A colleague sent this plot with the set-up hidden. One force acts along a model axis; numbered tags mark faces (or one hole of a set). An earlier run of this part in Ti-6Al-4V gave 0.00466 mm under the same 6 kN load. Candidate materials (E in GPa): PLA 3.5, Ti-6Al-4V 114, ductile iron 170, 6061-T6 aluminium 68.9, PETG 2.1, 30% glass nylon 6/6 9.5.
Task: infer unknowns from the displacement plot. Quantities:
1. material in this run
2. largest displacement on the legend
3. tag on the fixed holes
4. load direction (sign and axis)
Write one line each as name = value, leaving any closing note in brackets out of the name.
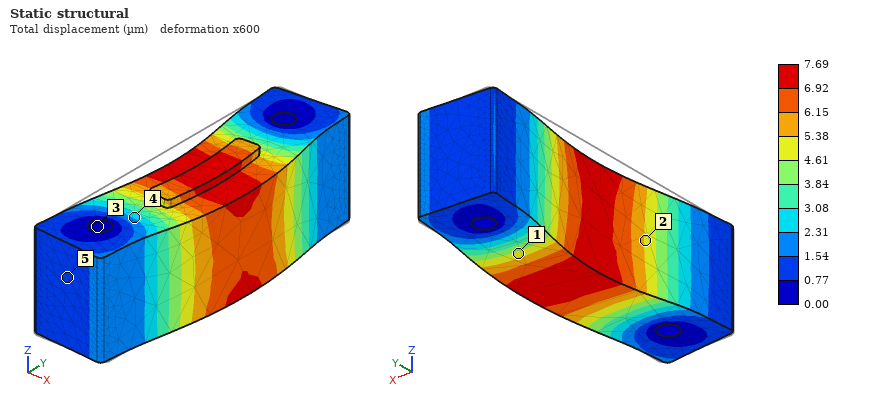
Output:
material in this run = 6061-T6 aluminium
largest displacement on the legend = 7.69 µm
tag on the fixed holes = 3
load direction = +X
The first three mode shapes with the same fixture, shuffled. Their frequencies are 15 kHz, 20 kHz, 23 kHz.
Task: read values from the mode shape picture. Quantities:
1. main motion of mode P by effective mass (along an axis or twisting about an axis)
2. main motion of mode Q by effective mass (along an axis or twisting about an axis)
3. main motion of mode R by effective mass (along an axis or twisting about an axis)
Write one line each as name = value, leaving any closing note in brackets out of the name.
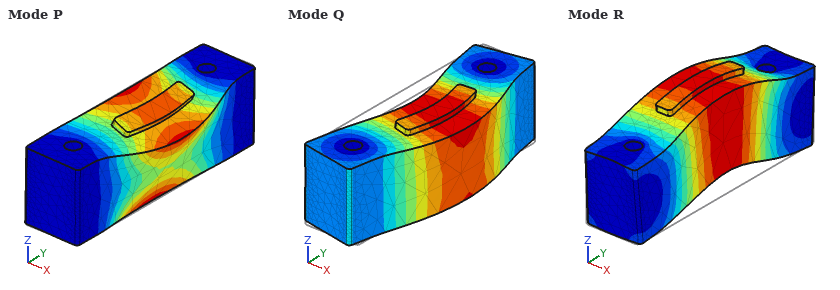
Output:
main motion of mode P by effective mass = twisting about Y
main motion of mode Q by effective mass = along X
main motion of mode R by effective mass = along Z
